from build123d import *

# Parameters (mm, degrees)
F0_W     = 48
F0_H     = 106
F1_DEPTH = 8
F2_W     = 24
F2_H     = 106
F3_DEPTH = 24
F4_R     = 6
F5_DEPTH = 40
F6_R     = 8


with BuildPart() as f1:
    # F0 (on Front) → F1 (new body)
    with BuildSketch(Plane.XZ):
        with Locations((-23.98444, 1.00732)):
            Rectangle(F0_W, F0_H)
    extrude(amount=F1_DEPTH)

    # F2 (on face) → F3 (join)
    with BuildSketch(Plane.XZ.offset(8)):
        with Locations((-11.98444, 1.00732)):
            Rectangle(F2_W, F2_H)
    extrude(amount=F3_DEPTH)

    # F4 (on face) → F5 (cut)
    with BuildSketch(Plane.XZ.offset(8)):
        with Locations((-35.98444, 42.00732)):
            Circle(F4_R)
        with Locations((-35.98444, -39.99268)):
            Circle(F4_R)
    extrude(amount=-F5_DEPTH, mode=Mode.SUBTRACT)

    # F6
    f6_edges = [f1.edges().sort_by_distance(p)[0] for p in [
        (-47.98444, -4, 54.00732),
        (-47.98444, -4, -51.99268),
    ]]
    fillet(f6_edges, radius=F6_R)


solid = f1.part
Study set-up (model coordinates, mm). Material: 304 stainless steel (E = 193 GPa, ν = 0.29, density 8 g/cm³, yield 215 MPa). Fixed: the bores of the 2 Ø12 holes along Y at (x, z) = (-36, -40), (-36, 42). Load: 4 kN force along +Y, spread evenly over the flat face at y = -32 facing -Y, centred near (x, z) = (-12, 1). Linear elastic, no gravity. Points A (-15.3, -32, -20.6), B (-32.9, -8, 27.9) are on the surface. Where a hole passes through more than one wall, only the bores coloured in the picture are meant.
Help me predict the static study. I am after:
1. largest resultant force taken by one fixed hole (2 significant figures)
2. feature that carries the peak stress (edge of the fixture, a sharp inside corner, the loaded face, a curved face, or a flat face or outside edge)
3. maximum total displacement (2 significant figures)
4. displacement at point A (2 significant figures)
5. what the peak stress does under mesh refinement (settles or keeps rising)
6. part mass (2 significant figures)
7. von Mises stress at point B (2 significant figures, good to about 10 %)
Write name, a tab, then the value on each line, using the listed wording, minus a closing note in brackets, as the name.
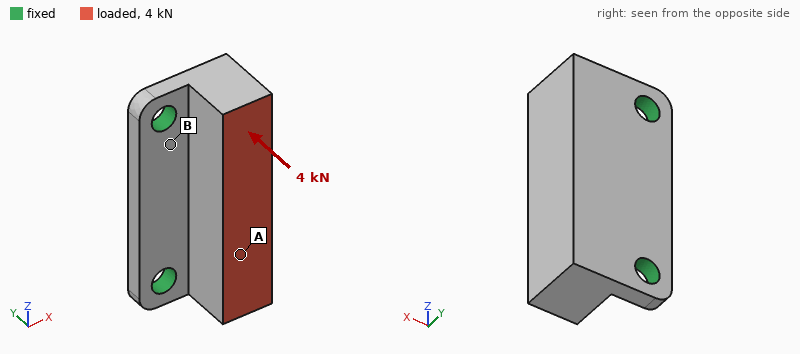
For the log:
largest resultant force taken by one fixed hole	2.0 kN
feature that carries the peak stress	edge of the fixture
maximum total displacement	49 µm
displacement at point A	37 µm
what the peak stress does under mesh refinement	keeps rising
part mass	800 g
von Mises stress at point B	38 MPa
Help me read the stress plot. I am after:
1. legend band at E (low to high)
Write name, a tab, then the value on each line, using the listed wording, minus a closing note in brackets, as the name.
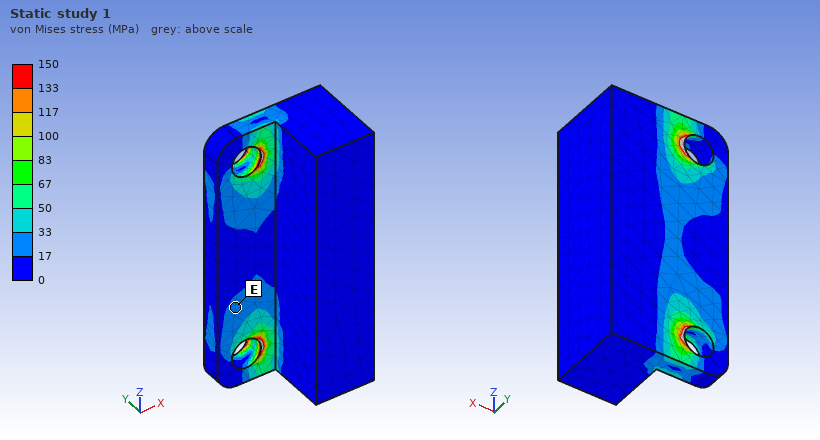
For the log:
legend band at E	17 to 33 MPa
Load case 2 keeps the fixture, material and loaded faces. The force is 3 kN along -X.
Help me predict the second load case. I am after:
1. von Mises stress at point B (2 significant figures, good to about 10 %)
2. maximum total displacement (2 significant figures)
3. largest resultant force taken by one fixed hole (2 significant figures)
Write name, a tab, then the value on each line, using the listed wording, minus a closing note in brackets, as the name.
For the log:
von Mises stress at point B	51 MPa
maximum total displacement	65 µm
largest resultant force taken by one fixed hole	1.5 kN
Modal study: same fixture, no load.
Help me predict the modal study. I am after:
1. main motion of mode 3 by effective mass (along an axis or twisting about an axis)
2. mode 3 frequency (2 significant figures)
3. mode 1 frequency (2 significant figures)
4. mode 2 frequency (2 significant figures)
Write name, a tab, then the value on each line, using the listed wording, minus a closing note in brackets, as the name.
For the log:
main motion of mode 3 by effective mass	along Y
mode 3 frequency	7700 Hz
mode 1 frequency	1900 Hz
mode 2 frequency	5900 Hz
